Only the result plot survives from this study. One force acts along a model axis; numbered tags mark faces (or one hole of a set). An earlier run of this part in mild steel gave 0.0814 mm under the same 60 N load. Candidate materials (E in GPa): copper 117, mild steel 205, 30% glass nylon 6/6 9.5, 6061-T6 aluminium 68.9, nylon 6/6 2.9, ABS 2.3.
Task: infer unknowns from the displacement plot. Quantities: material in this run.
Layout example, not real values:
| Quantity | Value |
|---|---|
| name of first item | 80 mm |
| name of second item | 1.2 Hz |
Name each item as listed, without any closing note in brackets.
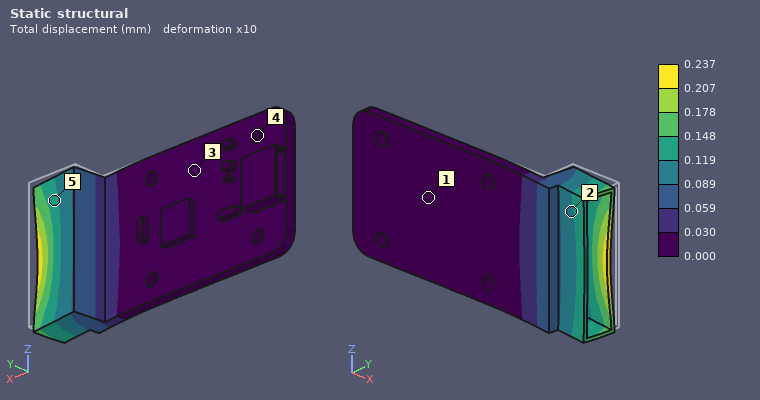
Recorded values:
| Quantity | Value |
|---|---|
| material in this run | 6061-T6 aluminium |
